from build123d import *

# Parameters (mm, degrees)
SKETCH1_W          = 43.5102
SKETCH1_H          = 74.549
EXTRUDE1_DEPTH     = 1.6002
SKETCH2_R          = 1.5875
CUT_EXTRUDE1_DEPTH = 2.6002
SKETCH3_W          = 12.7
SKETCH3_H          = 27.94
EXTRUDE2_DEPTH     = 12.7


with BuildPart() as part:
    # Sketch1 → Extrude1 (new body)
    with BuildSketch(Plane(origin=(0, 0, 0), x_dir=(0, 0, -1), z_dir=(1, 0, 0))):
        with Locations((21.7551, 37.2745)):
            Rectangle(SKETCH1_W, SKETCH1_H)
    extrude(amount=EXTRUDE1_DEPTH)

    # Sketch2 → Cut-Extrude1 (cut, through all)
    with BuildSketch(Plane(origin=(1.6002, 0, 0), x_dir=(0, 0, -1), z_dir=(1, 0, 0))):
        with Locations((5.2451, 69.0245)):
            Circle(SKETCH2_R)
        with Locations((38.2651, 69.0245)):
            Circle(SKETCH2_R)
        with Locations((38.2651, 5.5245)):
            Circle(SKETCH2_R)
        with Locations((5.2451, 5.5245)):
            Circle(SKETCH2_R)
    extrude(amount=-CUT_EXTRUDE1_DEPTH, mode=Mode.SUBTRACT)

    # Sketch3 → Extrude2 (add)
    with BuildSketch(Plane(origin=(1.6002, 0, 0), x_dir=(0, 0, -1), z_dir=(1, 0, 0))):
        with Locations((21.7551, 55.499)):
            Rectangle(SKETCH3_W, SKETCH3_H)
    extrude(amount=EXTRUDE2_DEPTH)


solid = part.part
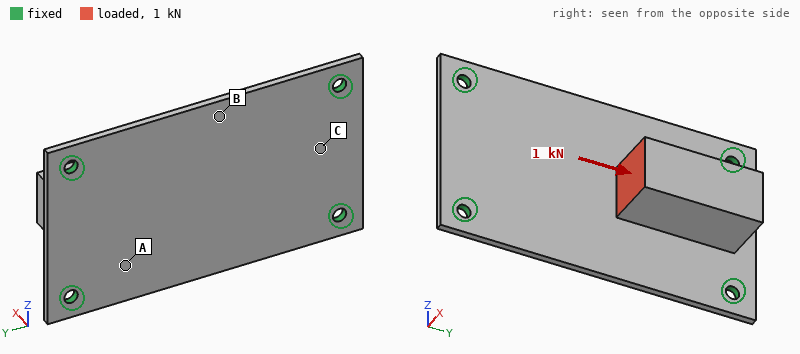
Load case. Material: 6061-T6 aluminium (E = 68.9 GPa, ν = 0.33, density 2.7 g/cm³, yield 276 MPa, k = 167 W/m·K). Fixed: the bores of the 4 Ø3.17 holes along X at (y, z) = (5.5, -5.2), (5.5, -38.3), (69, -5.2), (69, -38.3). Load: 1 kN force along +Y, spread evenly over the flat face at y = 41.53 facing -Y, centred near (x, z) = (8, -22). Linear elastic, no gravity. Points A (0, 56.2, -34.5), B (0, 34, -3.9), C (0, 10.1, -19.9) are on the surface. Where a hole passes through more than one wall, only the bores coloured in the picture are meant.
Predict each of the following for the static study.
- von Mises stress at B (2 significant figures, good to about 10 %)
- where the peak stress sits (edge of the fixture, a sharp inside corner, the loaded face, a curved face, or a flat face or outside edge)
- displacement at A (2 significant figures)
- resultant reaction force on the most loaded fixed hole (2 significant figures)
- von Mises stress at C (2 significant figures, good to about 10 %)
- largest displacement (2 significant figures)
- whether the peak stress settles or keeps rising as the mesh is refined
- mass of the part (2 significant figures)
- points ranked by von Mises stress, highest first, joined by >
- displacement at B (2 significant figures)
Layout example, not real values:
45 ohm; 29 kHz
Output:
65 MPa; edge of the fixture; 0.11 mm; 340 N; 34 MPa; 0.36 mm; keeps rising; 26 g; B > C > A; 0.27 mm
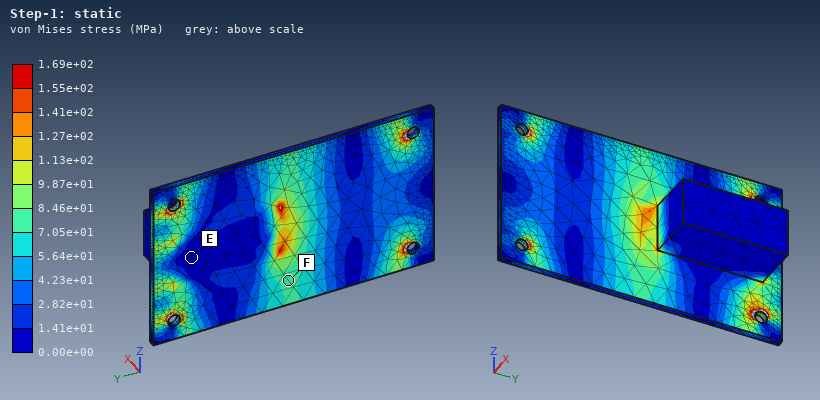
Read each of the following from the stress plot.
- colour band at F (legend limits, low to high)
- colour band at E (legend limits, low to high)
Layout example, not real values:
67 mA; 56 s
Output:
7.05e+01 to 8.46e+01 MPa; 0.00e+00 to 1.41e+01 MPa
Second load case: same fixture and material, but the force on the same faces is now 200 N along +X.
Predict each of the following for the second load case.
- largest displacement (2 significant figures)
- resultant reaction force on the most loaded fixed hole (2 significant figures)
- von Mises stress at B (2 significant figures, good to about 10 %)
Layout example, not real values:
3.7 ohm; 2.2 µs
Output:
0.27 mm; 64 N; 49 MPa
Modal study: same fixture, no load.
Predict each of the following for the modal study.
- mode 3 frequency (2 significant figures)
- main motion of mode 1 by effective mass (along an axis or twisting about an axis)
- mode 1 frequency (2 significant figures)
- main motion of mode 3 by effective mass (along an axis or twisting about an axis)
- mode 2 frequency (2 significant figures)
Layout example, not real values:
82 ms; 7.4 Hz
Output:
4600 Hz; along X; 1500 Hz; along X; 3600 Hz
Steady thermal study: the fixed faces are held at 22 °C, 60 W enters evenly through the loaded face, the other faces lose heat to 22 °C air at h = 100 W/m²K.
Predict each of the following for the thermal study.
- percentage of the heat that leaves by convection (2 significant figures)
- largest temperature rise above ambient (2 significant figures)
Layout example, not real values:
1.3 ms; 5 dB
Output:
35 %; 71 K
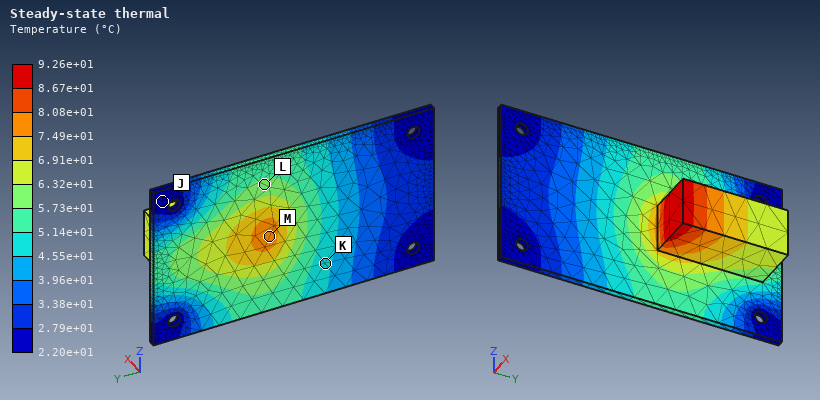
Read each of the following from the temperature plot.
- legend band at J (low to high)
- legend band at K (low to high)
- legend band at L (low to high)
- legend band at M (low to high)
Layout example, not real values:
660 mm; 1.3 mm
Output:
2.20e+01 to 2.79e+01 °C; 4.55e+01 to 5.14e+01 °C; 5.73e+01 to 6.32e+01 °C; 7.49e+01 to 8.08e+01 °C
